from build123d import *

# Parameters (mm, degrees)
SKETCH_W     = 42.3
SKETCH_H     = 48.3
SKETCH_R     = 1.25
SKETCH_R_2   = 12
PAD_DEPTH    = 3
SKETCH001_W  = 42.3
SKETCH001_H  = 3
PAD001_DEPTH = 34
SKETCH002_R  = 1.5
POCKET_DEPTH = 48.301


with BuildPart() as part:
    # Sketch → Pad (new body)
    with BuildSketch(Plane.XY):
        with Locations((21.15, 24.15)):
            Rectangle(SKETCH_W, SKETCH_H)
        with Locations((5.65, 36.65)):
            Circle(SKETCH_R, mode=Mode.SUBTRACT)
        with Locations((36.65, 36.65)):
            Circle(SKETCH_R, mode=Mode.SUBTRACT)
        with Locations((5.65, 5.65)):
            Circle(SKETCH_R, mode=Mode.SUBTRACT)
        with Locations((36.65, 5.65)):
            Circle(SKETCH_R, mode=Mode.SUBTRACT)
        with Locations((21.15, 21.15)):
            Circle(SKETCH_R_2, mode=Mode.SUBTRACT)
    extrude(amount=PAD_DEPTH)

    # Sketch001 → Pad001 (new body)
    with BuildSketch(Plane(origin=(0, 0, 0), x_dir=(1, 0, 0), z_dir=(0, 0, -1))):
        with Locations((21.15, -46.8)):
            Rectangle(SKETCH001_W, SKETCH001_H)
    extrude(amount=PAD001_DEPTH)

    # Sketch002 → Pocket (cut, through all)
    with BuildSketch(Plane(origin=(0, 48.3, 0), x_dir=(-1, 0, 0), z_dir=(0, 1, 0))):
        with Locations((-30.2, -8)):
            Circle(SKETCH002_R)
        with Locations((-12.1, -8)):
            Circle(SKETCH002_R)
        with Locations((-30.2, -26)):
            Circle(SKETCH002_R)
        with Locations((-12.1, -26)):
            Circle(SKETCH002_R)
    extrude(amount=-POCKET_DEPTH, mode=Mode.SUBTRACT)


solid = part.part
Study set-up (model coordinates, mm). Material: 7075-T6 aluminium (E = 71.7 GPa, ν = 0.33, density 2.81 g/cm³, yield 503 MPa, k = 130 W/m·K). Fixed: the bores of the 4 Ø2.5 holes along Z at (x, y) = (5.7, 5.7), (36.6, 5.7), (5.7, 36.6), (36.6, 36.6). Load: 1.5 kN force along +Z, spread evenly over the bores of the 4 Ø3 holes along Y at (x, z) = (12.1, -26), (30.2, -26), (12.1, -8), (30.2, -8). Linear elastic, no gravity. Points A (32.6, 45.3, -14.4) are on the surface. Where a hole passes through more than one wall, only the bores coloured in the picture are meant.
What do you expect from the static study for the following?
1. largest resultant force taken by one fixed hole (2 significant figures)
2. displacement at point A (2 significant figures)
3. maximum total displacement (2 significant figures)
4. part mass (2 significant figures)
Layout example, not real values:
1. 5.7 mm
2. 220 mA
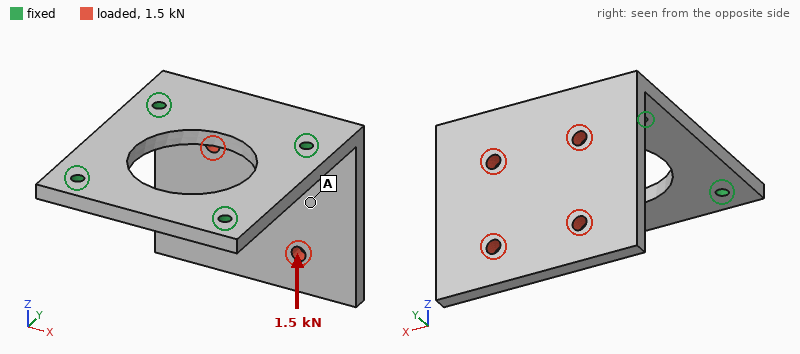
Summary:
1. 790 N
2. 0.25 mm
3. 0.54 mm
4. 25 g
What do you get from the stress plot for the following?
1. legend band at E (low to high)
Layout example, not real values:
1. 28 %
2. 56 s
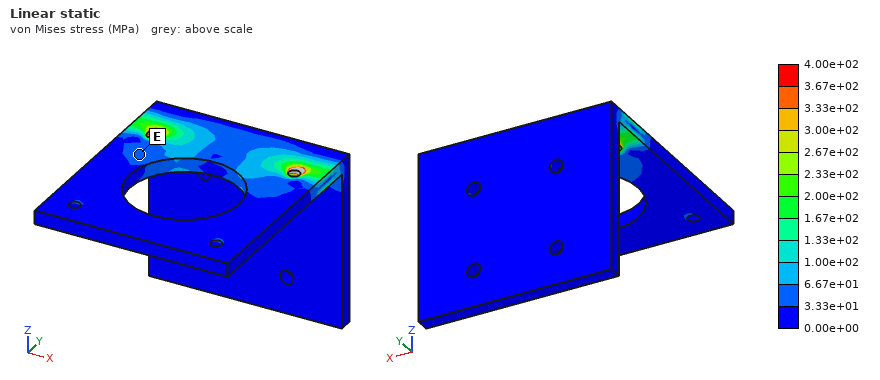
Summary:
1. 3.33e+01 to 6.67e+01 MPa
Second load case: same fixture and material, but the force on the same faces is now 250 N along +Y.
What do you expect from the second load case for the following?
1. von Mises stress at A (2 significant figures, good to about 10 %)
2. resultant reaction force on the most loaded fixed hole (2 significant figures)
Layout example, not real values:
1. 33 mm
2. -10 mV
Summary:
1. 22 MPa
2. 130 N
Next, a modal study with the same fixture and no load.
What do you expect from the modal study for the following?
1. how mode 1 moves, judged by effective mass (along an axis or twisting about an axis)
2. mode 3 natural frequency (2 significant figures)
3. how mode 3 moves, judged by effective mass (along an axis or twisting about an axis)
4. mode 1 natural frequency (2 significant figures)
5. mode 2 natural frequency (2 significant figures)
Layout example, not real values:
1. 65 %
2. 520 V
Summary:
1. along Y
2. 4900 Hz
3. along X
4. 1300 Hz
5. 3300 Hz
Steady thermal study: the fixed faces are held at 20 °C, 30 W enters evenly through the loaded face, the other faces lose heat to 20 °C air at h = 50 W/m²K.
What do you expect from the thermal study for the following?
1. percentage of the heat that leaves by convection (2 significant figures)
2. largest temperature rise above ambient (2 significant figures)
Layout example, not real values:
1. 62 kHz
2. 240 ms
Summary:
1. 23 %
2. 50 K
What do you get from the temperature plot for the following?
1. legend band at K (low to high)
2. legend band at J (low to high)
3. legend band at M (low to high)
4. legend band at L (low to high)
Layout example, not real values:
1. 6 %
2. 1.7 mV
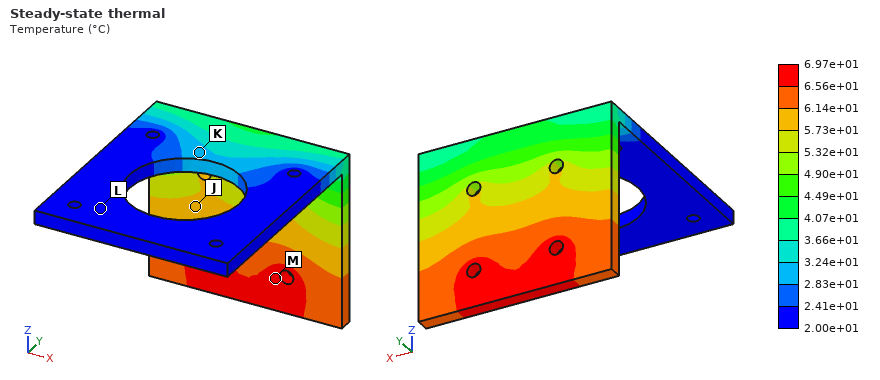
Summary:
1. 2.83e+01 to 3.24e+01 °C
2. 5.73e+01 to 6.14e+01 °C
3. 6.56e+01 to 6.97e+01 °C
4. 2.00e+01 to 2.41e+01 °C
